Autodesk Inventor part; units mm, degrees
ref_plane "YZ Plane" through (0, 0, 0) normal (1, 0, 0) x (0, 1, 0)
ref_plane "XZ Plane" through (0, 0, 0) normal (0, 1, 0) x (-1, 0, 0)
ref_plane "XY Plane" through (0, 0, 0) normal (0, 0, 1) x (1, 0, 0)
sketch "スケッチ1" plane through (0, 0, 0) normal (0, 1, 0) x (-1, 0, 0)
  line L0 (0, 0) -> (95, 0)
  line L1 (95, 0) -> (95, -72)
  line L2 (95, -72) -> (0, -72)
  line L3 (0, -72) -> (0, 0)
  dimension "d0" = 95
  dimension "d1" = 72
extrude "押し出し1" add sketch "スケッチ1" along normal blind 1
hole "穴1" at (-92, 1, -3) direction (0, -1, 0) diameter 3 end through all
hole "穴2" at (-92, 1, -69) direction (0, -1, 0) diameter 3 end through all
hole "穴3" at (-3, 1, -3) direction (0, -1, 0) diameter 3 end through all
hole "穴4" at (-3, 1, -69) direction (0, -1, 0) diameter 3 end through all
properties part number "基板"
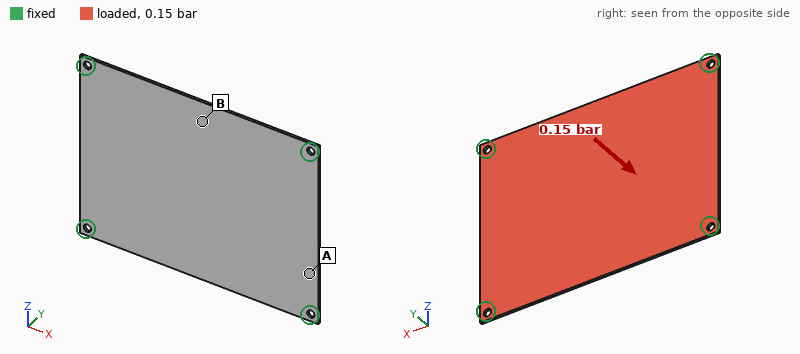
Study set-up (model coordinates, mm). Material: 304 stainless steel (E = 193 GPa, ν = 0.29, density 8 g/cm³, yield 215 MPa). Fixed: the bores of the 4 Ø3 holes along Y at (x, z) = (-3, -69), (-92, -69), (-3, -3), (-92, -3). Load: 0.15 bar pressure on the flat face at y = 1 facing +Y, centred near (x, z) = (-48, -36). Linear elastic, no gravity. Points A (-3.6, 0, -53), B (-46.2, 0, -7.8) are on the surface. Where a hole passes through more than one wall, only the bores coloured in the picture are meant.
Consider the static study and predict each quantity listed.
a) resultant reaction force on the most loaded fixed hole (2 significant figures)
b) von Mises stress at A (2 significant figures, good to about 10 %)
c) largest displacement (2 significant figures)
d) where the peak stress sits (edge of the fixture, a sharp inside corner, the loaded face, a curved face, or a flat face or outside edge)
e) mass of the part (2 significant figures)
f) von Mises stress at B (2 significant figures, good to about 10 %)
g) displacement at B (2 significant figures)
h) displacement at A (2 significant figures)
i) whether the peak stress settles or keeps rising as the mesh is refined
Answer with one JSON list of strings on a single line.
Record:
["26 N", "15 MPa", "0.29 mm", "edge of the fixture", "54 g", "40 MPa", "0.25 mm", "0.045 mm", "keeps rising"]
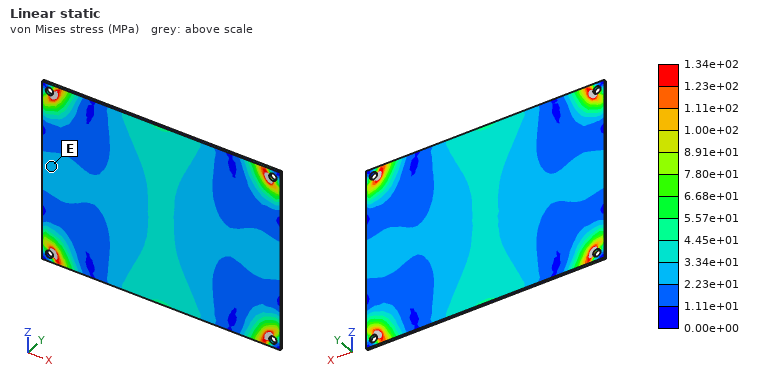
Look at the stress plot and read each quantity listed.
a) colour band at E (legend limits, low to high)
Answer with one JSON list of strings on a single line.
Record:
["2.23e+01 to 3.34e+01 MPa"]
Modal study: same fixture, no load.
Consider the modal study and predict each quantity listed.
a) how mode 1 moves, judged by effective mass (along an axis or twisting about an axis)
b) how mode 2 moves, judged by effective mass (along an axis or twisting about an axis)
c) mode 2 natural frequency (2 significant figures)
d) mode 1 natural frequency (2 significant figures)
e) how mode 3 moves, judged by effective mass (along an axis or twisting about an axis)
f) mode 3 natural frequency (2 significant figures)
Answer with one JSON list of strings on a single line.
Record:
["along Y", "twisting about X", "810 Hz", "470 Hz", "twisting about Z", "1100 Hz"]
